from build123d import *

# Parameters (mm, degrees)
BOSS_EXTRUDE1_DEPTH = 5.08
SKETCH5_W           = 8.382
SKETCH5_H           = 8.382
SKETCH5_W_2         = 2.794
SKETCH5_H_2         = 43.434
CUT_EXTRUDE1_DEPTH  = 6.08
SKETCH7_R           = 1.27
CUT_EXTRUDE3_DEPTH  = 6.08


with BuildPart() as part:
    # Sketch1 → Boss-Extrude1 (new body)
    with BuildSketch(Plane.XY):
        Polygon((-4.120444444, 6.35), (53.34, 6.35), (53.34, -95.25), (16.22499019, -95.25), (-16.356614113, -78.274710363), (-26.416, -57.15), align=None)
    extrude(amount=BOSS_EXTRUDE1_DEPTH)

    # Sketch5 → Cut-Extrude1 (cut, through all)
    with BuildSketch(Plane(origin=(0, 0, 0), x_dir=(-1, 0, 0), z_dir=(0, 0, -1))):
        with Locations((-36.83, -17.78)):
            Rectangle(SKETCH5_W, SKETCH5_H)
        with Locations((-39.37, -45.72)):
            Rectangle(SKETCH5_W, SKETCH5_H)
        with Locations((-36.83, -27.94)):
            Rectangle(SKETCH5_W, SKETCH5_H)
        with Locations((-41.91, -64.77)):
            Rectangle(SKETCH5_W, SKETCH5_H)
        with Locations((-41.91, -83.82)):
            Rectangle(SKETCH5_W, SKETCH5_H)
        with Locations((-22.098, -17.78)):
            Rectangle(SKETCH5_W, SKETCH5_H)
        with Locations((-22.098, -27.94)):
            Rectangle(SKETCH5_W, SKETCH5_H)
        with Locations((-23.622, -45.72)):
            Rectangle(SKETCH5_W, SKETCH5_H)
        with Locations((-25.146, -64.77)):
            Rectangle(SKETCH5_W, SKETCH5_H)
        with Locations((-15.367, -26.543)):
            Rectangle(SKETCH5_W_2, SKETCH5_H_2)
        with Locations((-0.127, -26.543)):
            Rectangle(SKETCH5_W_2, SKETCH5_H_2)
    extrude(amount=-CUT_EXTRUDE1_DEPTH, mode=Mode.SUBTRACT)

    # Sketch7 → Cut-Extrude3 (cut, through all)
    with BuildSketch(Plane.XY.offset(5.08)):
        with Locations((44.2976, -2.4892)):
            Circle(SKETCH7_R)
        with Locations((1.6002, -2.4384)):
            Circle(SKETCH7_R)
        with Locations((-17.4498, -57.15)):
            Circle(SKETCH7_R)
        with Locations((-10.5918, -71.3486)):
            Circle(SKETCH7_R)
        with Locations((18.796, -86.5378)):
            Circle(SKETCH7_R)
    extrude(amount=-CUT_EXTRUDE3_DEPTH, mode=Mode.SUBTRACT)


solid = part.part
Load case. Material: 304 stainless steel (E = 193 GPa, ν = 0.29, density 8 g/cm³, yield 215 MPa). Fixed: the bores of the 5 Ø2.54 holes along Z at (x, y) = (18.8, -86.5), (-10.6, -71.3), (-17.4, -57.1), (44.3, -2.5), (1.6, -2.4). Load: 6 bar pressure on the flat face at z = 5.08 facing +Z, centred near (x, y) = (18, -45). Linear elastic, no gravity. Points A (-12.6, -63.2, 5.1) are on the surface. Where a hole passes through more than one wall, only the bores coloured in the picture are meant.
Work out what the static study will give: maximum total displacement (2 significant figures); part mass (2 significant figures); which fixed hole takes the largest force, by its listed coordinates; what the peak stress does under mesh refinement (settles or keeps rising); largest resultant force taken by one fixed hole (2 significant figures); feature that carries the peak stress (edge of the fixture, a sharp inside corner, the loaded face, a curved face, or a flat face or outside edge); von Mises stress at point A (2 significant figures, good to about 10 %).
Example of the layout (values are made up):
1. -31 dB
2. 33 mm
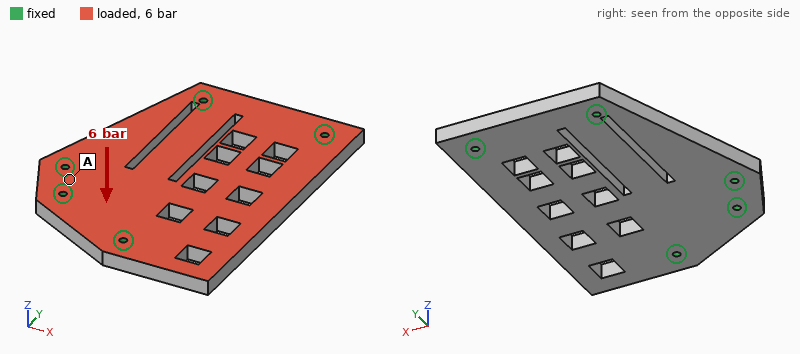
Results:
1. 0.10 mm
2. 240 g
3. (18.8, -86.5)
4. keeps rising
5. 1.2 kN
6. edge of the fixture
7. 33 MPa
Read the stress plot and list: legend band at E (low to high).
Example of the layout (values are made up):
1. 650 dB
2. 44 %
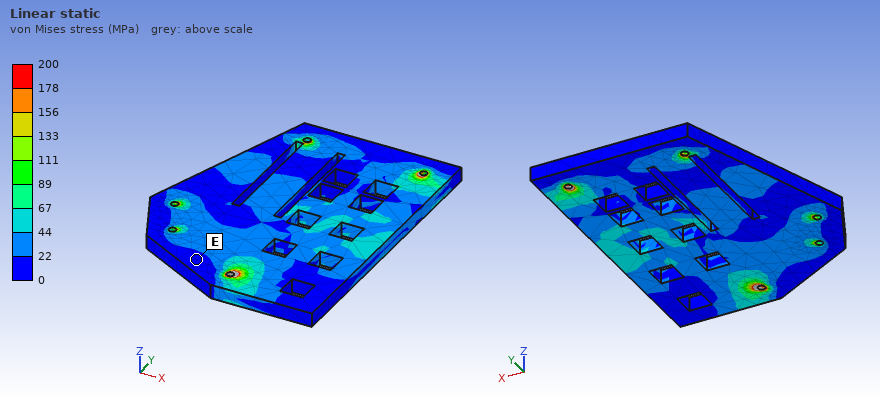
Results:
1. 0 to 22 MPa
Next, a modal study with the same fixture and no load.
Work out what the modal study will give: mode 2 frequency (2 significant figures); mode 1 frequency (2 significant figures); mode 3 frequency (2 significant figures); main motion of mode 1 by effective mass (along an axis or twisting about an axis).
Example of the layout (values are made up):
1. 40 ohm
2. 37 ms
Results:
1. 4100 Hz
2. 2500 Hz
3. 5600 Hz
4. along Z
